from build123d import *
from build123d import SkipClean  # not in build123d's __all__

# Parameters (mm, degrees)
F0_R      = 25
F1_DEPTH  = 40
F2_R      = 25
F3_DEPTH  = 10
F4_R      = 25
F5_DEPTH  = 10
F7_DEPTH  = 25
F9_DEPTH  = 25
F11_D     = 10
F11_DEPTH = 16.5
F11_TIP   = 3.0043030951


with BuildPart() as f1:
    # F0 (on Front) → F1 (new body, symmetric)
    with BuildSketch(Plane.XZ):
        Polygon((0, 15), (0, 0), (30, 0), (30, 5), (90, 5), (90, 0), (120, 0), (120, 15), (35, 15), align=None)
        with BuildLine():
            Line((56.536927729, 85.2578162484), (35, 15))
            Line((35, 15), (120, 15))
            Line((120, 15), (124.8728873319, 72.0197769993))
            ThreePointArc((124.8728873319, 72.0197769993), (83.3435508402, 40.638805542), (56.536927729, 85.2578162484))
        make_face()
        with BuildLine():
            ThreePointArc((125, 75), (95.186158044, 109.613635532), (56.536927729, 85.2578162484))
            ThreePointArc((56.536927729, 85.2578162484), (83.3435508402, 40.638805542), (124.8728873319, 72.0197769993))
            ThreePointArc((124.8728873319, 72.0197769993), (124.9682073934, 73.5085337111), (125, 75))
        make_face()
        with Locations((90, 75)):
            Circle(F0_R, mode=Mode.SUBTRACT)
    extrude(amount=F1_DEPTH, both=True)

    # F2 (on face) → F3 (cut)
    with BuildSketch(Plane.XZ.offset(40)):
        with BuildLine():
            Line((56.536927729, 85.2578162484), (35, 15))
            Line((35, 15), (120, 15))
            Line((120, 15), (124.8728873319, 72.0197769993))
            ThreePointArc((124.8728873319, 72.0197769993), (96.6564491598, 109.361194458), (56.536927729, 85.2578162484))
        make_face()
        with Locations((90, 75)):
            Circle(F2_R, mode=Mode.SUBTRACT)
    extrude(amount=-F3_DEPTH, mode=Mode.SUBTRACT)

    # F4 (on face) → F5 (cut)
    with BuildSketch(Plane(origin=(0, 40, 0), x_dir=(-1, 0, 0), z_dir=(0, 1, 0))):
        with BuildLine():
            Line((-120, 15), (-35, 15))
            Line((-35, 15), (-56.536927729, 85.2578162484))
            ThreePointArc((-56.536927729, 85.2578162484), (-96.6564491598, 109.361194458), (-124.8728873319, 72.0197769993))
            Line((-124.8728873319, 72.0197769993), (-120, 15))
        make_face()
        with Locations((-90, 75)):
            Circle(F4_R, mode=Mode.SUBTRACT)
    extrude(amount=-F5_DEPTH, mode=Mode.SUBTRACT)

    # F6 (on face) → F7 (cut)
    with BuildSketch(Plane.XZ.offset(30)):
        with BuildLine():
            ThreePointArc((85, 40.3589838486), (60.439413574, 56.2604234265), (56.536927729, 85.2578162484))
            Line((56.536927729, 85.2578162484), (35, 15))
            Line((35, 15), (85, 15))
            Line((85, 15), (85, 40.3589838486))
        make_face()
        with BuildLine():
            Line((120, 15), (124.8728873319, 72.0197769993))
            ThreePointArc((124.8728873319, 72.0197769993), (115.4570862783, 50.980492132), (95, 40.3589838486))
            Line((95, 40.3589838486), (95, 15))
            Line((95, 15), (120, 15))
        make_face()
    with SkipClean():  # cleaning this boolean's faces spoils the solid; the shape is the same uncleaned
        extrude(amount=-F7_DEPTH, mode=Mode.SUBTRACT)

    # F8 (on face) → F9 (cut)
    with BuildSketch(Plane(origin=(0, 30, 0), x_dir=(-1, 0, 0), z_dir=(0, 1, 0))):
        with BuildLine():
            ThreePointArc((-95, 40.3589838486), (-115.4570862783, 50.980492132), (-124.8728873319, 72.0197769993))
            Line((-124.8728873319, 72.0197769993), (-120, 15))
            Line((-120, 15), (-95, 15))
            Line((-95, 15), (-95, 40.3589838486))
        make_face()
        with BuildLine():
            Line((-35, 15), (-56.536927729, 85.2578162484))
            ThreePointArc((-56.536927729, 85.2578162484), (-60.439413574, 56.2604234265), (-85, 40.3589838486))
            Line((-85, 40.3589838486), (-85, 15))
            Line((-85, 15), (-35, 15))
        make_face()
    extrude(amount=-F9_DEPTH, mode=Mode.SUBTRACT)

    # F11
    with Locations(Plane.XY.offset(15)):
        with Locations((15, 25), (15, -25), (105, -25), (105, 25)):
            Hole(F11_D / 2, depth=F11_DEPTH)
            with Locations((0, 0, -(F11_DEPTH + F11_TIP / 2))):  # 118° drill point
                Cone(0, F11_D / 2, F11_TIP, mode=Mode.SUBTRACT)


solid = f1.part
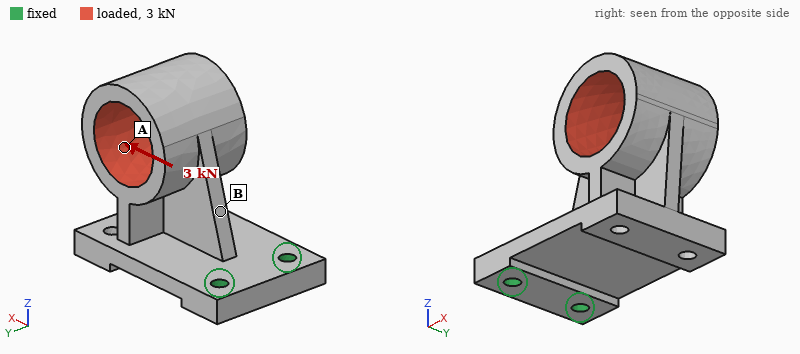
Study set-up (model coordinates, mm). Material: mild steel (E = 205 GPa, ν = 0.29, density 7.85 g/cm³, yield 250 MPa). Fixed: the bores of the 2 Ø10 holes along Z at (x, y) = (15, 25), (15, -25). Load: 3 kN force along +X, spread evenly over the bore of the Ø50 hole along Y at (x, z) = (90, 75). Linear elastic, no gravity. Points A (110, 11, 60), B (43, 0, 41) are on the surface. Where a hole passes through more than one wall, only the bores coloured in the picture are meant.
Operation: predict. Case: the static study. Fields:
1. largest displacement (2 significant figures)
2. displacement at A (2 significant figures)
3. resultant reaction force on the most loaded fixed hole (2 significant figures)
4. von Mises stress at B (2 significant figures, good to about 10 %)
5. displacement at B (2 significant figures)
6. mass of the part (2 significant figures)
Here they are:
0.44 mm
0.32 mm
1.7 kN
31 MPa
0.12 mm
2.1 kg
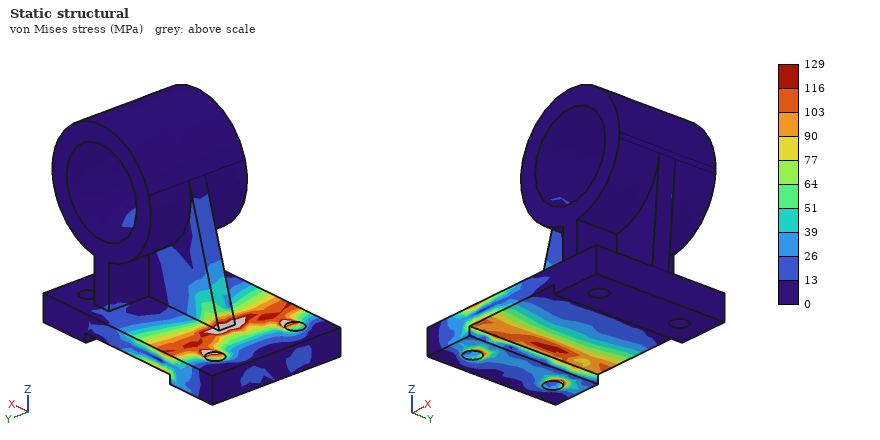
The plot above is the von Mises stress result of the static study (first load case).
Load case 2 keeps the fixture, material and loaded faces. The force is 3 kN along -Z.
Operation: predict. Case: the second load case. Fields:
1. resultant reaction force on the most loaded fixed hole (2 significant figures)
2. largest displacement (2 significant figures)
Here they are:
1.5 kN
0.37 mm
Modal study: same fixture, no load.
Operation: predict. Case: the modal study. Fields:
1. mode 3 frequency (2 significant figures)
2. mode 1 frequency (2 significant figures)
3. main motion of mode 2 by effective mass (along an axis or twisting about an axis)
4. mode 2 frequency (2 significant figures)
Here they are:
2500 Hz
370 Hz
along Y
600 Hz
